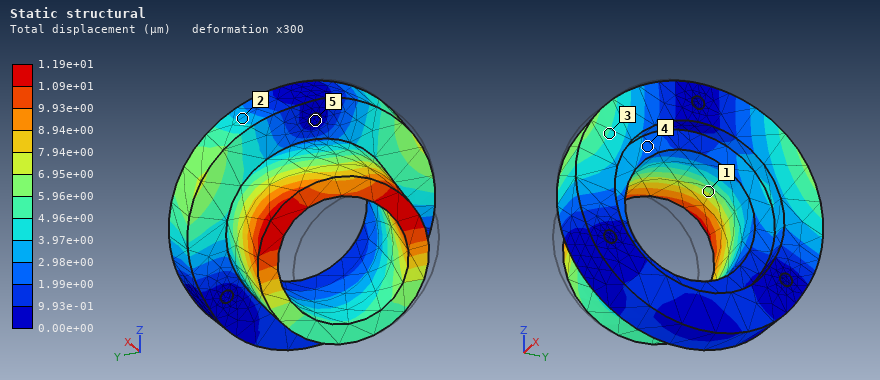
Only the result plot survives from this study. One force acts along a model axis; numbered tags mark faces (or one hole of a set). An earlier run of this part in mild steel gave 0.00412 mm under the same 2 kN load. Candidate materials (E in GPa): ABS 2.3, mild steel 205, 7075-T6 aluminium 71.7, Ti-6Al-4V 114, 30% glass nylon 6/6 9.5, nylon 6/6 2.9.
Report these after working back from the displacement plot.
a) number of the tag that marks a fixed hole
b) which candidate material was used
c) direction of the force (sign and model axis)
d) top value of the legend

5
7075-T6 aluminium
+Y
1.19e+01 µm
